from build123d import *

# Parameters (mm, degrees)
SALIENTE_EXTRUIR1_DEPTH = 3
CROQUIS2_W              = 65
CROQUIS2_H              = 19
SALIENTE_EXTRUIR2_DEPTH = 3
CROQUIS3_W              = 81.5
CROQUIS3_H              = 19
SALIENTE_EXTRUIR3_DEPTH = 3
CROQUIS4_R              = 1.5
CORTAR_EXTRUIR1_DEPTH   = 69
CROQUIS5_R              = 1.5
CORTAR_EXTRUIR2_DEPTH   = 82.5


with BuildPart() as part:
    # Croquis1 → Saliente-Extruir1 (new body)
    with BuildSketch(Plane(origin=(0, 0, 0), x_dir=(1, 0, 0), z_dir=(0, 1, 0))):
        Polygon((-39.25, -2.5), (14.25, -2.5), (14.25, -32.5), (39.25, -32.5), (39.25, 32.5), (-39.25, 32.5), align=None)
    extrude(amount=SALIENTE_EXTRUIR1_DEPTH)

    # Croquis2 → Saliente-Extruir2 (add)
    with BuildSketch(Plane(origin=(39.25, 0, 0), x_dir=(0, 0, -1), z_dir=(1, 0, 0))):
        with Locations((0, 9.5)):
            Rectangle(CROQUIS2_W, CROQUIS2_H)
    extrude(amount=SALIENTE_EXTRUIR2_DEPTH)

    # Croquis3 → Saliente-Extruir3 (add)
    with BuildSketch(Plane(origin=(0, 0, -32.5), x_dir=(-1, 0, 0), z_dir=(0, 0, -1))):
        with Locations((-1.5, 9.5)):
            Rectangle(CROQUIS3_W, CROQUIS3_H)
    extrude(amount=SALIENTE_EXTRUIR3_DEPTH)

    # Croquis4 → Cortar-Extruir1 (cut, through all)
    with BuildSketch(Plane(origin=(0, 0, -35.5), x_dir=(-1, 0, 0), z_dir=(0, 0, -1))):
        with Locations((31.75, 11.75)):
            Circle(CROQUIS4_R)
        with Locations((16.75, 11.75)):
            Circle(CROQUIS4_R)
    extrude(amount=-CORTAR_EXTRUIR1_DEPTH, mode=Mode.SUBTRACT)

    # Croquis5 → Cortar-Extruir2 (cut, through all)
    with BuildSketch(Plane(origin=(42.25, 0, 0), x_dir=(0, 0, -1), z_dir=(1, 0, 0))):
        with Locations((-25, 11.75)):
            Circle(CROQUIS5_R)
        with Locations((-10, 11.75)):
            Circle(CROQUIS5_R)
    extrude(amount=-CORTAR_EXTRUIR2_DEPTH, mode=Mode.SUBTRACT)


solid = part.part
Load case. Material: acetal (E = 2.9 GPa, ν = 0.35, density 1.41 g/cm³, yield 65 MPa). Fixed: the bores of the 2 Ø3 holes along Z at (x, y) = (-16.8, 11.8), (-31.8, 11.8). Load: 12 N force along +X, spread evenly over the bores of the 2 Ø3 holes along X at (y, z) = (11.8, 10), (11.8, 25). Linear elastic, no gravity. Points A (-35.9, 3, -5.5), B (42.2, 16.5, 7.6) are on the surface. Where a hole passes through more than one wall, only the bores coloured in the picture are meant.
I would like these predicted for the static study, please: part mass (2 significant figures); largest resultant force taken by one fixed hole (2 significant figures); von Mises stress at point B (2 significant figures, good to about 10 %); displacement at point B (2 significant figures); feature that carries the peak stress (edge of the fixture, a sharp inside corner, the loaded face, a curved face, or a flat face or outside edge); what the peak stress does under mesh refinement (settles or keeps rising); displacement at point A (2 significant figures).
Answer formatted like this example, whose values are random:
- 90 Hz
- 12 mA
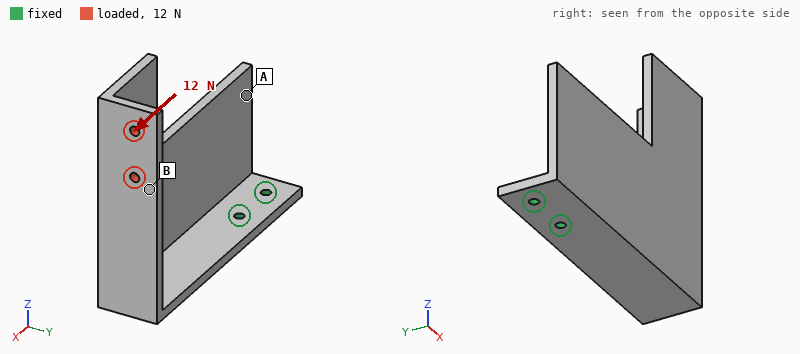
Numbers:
- 26 g
- 32 N
- 1.3 MPa
- 0.72 mm
- edge of the fixture
- keeps rising
- 0.20 mm
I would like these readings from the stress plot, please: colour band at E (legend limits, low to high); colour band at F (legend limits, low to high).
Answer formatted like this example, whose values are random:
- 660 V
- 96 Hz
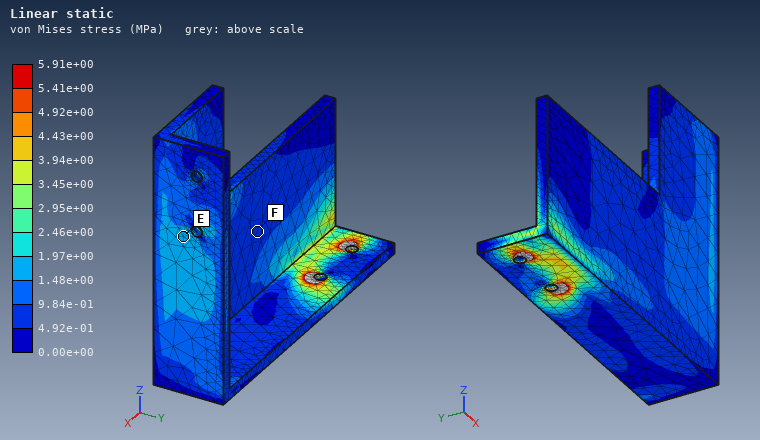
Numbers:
- 1.48e+00 to 1.97e+00 MPa
- 4.92e-01 to 9.84e-01 MPa
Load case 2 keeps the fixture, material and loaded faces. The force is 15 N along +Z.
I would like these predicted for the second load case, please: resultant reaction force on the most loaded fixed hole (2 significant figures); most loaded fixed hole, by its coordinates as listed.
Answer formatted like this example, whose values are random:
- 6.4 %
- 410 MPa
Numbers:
- 55 N
- (-16.8, 11.8)
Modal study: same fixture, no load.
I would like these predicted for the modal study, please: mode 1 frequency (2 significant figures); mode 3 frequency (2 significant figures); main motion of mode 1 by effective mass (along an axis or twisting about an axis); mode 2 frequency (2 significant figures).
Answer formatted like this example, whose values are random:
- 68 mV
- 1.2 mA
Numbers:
- 100 Hz
- 450 Hz
- along Y
- 200 Hz
